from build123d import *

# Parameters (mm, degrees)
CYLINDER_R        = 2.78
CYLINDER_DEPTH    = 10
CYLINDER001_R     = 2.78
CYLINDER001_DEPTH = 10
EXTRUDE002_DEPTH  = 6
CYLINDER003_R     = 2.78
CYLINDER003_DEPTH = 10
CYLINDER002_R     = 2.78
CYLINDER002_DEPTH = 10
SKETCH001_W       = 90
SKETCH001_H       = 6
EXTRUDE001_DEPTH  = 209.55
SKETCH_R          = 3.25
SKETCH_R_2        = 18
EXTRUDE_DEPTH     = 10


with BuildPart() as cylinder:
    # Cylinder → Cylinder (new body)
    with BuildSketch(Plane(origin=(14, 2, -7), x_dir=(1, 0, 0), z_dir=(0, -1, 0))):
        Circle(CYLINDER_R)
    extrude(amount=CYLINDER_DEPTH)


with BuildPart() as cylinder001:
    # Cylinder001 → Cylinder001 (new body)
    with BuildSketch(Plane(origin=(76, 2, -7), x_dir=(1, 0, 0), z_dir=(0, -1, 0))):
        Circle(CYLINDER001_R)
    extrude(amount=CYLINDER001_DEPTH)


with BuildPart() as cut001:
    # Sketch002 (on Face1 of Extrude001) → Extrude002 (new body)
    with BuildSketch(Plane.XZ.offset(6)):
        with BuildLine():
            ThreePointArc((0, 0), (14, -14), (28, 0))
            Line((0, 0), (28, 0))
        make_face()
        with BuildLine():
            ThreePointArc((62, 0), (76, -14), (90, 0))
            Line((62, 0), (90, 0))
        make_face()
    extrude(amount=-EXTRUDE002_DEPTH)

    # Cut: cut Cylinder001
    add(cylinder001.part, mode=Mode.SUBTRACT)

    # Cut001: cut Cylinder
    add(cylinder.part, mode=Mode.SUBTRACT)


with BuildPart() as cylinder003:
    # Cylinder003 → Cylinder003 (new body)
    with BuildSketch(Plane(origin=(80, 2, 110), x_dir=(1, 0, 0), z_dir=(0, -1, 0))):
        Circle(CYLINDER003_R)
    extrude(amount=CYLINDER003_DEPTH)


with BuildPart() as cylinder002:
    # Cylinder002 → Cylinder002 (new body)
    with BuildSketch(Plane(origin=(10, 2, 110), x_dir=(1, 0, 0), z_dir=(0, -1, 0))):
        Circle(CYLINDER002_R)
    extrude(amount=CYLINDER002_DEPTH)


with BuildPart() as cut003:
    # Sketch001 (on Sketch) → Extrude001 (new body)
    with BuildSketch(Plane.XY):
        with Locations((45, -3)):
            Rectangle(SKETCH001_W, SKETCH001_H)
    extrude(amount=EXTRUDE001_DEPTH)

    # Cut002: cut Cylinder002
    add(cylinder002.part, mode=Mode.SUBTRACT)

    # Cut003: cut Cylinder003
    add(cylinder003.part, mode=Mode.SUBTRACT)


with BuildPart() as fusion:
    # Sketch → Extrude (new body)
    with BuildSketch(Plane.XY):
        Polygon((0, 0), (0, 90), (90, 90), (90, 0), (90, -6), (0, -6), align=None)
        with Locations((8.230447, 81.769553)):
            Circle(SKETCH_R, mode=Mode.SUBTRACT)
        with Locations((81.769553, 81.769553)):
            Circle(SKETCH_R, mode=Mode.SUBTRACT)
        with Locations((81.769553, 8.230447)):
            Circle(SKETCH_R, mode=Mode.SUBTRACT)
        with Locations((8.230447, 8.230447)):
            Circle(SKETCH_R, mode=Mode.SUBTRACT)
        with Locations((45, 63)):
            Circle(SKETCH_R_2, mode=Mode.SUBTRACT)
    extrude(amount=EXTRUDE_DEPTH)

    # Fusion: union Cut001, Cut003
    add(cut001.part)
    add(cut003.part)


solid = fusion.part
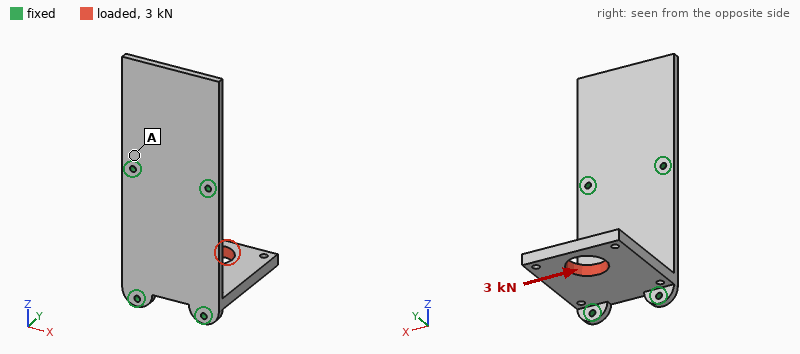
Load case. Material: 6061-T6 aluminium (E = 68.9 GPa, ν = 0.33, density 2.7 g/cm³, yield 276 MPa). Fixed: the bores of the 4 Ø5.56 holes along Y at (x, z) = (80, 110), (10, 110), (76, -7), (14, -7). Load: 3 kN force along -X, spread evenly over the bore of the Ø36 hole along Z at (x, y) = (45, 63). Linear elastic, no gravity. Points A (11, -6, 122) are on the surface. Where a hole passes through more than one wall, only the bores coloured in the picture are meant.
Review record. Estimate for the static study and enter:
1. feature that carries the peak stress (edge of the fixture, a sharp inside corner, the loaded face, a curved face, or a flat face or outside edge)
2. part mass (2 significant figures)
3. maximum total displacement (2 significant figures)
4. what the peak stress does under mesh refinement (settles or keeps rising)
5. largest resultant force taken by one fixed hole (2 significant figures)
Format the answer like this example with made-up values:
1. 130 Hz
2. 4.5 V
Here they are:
1. edge of the fixture
2. 500 g
3. 0.14 mm
4. keeps rising
5. 3.3 kN
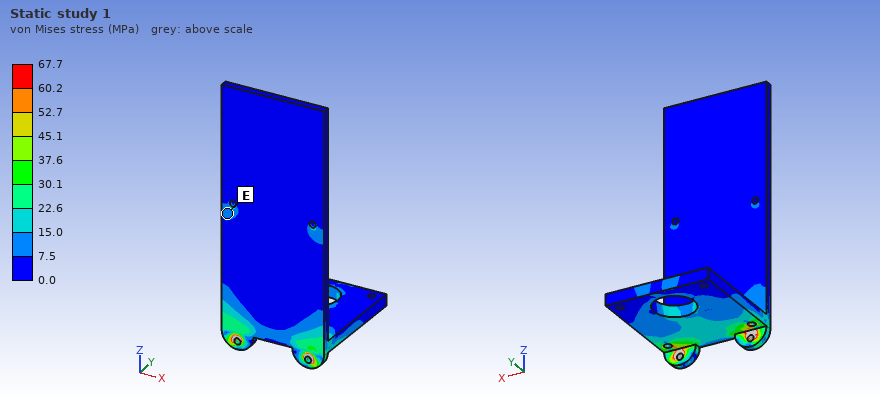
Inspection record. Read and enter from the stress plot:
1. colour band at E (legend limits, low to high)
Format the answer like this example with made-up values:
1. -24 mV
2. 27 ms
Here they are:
1. 7.5 to 15.0 MPa
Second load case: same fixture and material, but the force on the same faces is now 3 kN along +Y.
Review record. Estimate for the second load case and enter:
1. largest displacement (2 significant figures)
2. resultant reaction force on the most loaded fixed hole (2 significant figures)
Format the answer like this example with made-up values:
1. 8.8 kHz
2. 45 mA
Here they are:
1. 0.16 mm
2. 1.4 kN
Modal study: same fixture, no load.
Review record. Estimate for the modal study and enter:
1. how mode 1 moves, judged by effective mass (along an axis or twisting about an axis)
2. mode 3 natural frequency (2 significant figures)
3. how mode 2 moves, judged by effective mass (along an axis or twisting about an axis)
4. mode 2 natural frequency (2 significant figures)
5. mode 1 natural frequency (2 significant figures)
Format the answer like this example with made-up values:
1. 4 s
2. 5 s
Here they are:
1. along Y
2. 1300 Hz
3. along Z
4. 620 Hz
5. 460 Hz
